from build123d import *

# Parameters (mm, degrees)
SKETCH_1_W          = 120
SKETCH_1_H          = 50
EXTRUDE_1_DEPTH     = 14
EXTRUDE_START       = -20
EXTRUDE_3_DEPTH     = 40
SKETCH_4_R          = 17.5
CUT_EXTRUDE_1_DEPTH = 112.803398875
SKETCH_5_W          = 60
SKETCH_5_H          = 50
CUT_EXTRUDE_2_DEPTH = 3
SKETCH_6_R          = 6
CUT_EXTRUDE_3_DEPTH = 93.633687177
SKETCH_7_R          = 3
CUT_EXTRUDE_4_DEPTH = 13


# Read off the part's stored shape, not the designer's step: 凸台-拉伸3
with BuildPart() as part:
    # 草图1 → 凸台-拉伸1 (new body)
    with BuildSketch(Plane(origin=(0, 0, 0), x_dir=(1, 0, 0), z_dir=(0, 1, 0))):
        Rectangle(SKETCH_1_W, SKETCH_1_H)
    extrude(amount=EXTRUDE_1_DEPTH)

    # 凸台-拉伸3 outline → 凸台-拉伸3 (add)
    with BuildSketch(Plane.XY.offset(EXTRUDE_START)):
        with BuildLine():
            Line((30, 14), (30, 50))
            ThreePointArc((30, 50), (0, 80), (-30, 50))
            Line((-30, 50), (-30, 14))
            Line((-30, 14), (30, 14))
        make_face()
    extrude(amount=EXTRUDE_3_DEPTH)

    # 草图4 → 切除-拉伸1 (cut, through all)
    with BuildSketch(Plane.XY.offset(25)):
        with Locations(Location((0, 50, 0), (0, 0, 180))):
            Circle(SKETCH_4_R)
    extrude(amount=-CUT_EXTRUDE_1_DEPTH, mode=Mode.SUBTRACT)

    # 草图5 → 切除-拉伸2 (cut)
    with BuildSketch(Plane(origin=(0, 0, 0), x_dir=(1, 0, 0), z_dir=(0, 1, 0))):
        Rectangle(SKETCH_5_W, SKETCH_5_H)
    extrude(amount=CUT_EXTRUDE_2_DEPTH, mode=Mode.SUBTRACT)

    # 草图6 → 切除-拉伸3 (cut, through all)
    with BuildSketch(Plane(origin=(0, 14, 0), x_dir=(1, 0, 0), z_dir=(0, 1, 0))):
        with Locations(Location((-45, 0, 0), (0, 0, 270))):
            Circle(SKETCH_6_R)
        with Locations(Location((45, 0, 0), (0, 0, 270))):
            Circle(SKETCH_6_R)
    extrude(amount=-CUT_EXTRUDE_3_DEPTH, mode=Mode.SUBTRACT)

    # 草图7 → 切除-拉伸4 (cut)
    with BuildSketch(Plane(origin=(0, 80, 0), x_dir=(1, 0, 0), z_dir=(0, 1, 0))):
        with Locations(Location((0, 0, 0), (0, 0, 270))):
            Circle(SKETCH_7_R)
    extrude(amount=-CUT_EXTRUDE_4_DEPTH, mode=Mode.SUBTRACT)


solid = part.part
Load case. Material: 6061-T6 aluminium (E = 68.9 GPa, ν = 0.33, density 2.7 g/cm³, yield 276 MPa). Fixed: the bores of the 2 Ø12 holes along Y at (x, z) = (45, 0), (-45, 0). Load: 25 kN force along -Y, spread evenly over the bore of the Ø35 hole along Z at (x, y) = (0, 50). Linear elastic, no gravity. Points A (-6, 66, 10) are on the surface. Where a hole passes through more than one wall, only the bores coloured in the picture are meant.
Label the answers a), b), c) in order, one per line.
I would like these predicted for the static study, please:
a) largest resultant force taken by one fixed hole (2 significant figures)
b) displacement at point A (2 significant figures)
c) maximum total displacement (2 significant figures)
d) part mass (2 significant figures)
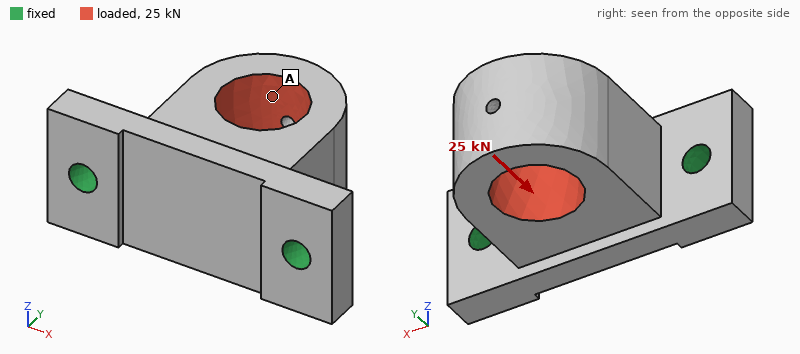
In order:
a) 14 kN
b) 51 µm
c) 52 µm
d) 480 g
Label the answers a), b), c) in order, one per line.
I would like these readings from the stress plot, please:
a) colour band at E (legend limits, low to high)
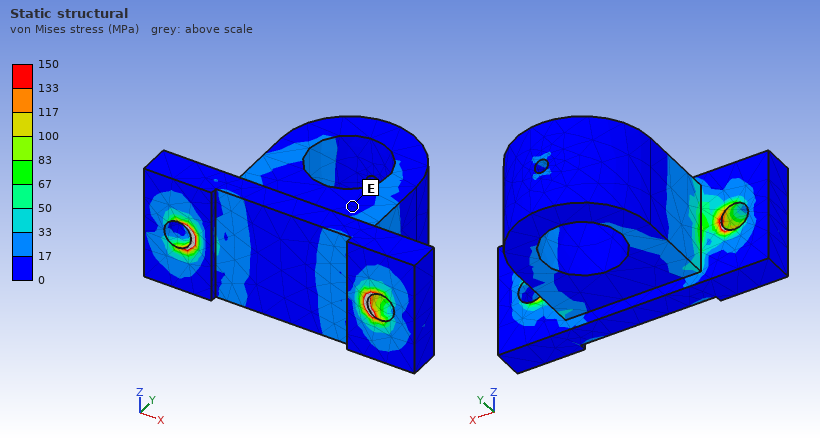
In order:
a) 0 to 17 MPa
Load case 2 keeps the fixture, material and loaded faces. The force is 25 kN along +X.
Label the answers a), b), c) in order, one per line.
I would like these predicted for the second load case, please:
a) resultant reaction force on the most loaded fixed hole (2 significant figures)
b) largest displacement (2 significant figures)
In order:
a) 19 kN
b) 0.17 mm
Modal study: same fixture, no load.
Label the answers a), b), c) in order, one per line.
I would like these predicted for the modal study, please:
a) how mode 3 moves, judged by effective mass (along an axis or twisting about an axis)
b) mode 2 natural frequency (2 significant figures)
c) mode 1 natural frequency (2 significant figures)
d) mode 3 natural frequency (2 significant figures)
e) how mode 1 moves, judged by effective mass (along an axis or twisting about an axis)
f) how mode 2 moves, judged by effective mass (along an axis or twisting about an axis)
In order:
a) along Y
b) 4800 Hz
c) 2200 Hz
d) 6500 Hz
e) along Z
f) along X
